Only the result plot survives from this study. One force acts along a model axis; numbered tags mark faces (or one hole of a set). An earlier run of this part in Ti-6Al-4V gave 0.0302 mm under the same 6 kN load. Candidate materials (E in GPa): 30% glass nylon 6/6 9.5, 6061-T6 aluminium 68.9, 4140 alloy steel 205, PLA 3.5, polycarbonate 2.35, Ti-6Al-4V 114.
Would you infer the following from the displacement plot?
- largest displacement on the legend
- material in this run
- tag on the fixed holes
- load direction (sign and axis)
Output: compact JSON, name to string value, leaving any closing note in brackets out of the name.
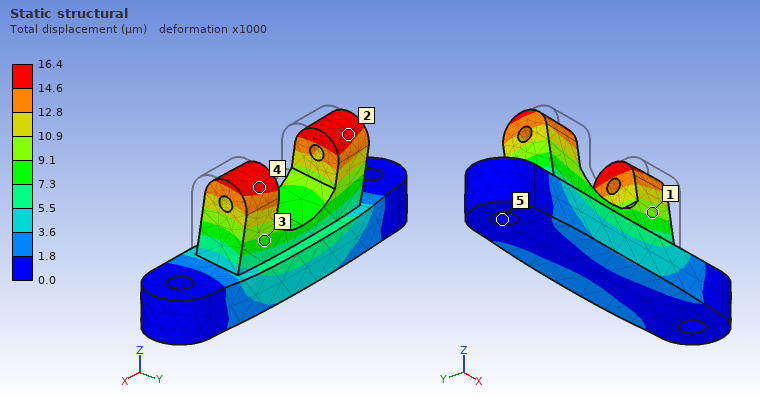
{"largest displacement on the legend": "16.4 µm", "material in this run": "4140 alloy steel", "tag on the fixed holes": "5", "load direction": "+Y"}
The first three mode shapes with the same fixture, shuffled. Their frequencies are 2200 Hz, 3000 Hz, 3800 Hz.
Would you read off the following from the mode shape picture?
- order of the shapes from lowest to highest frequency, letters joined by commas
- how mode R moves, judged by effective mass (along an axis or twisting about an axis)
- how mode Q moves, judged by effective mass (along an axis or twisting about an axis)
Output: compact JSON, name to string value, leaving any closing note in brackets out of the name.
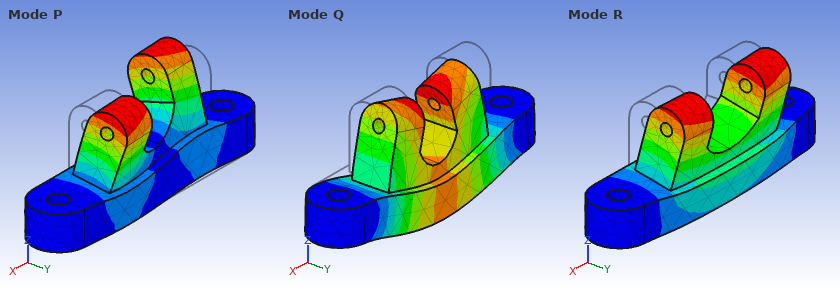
{"order of the shapes from lowest to highest frequency, letters joined by commas": "R, Q, P", "how mode R moves, judged by effective mass": "along Y", "how mode Q moves, judged by effective mass": "along Z"}
